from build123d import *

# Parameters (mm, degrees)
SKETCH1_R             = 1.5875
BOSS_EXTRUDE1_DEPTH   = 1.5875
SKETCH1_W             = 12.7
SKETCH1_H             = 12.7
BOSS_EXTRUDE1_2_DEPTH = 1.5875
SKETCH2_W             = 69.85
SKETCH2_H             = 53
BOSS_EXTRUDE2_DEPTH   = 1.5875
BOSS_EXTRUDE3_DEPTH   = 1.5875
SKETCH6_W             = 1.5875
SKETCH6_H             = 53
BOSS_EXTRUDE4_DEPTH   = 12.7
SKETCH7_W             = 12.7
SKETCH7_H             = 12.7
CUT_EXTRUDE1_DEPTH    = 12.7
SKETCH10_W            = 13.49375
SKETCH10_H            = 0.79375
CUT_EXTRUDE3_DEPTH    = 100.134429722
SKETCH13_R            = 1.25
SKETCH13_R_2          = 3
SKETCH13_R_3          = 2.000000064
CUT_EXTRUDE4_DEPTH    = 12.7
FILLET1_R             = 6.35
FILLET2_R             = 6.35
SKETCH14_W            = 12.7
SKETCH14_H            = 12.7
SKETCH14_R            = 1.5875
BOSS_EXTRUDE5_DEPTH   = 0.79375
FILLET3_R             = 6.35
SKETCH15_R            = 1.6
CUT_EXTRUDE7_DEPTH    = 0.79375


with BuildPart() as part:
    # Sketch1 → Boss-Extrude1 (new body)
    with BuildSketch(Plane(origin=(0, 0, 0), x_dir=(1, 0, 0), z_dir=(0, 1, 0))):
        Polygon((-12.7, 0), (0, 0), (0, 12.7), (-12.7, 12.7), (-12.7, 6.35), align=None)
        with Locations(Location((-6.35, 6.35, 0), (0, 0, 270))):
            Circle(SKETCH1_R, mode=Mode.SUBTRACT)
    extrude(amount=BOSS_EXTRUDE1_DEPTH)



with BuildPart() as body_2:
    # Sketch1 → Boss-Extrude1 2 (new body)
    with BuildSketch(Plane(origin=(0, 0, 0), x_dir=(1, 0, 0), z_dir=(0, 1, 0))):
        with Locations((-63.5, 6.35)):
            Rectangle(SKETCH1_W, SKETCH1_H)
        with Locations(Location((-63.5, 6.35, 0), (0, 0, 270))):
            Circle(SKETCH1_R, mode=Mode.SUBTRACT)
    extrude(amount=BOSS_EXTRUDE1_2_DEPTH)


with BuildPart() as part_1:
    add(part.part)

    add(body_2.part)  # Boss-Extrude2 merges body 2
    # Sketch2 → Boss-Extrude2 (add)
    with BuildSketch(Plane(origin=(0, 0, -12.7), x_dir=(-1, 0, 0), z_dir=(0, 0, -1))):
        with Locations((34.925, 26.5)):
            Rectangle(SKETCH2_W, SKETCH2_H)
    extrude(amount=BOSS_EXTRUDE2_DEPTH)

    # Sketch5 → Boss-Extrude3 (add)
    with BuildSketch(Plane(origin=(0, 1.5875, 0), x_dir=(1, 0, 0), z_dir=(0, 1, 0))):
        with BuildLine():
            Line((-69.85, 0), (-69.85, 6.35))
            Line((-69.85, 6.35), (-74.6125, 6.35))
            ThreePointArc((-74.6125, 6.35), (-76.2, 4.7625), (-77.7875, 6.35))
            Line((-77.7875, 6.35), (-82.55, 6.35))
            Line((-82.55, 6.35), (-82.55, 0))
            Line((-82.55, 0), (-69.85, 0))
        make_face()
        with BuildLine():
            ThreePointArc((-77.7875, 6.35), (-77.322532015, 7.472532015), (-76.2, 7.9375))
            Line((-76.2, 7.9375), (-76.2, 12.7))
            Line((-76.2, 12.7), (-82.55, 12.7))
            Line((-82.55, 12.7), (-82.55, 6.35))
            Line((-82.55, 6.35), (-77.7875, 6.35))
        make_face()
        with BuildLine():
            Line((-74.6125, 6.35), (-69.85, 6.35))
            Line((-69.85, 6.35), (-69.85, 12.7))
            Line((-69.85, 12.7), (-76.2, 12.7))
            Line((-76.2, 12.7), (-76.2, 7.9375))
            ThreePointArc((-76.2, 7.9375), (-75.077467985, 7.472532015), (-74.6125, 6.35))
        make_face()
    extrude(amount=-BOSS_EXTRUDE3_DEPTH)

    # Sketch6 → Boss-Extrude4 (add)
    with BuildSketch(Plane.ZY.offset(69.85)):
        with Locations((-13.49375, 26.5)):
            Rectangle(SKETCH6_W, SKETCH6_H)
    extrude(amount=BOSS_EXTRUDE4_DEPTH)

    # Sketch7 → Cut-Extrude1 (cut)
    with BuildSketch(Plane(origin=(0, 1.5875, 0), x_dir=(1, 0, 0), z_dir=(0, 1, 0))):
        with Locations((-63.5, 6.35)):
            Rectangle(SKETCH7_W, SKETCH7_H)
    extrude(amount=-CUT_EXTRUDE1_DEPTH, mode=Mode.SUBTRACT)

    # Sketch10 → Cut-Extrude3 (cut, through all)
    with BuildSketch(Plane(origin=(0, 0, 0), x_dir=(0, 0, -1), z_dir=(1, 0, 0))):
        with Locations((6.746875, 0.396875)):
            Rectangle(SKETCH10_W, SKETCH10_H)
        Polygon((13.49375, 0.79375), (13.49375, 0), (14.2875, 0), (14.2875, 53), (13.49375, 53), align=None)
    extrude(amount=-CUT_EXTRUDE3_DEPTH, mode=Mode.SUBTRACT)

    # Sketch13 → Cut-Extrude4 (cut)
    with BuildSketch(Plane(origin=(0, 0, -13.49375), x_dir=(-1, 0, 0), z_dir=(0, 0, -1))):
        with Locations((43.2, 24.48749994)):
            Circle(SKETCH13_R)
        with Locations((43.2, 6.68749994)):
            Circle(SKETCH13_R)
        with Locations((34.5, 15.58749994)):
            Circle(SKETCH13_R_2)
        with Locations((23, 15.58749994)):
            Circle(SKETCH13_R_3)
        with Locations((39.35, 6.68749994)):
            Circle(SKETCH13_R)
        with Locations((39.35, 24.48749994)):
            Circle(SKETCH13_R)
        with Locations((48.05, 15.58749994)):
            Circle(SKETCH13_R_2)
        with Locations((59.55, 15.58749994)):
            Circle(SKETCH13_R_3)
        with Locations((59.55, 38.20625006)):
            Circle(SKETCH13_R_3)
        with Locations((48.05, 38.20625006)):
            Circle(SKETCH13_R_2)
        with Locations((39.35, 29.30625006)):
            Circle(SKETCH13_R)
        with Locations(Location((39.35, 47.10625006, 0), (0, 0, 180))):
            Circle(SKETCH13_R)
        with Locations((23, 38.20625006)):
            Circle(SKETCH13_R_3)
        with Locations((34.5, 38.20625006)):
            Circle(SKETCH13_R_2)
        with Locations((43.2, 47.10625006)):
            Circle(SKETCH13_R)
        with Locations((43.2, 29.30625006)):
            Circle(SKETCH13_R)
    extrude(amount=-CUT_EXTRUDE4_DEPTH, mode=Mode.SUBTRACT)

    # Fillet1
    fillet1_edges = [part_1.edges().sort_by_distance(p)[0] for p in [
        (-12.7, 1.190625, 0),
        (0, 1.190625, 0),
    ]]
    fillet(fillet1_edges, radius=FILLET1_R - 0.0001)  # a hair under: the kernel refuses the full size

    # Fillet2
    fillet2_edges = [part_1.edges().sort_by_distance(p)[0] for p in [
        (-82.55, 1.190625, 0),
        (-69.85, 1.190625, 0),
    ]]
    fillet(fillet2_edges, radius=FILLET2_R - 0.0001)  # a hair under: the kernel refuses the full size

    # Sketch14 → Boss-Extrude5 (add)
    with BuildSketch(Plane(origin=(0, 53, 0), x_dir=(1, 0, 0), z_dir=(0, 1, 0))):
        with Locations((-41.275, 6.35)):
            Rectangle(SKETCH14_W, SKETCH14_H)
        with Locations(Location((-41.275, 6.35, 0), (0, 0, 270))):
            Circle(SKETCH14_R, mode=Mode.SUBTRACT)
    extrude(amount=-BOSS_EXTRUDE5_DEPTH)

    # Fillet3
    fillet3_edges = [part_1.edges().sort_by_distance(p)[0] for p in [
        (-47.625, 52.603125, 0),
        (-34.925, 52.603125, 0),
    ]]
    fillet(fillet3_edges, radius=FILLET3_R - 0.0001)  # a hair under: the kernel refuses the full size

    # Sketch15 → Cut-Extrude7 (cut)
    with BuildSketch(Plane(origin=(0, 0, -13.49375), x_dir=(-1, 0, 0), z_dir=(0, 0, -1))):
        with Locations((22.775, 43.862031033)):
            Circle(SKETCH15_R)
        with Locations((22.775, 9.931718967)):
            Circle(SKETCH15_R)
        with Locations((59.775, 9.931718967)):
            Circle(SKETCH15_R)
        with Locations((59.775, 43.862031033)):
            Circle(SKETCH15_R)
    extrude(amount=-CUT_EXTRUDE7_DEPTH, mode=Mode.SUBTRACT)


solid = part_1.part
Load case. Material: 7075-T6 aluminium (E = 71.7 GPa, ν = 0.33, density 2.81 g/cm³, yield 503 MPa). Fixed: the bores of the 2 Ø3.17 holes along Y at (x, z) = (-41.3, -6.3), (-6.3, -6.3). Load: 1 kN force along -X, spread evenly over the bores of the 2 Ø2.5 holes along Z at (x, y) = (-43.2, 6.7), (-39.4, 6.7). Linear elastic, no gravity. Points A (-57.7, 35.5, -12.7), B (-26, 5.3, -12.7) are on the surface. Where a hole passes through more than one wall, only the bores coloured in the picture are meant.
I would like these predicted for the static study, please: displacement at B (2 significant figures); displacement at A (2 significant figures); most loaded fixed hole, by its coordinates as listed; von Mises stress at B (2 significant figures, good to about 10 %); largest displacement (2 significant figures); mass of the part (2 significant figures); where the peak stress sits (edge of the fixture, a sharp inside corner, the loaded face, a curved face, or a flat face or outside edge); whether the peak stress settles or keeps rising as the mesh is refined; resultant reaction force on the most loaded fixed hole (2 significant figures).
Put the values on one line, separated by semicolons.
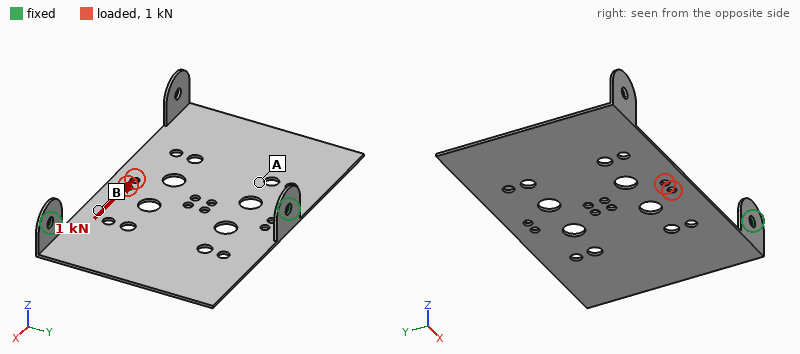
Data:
0.17 mm; 0.095 mm; (-6.3, -6.3); 120 MPa; 0.34 mm; 10.0 g; edge of the fixture; keeps rising; 880 N
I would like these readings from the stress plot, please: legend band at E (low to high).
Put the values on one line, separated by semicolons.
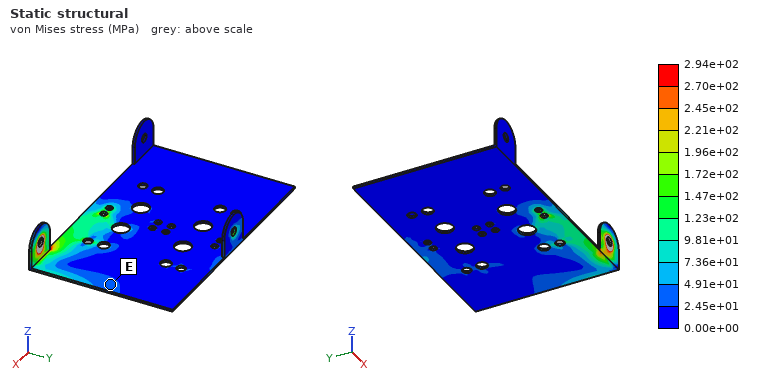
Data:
2.45e+01 to 4.91e+01 MPa
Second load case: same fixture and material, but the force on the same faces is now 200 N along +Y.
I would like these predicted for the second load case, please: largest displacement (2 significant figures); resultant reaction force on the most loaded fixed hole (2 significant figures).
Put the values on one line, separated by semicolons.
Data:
0.95 mm; 120 N
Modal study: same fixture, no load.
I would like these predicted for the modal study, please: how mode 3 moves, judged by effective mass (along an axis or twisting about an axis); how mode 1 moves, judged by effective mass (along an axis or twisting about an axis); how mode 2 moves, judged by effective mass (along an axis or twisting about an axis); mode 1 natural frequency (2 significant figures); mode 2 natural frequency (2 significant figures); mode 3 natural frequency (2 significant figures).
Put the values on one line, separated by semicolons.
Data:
along Z; along Z; twisting about X; 170 Hz; 550 Hz; 600 Hz
